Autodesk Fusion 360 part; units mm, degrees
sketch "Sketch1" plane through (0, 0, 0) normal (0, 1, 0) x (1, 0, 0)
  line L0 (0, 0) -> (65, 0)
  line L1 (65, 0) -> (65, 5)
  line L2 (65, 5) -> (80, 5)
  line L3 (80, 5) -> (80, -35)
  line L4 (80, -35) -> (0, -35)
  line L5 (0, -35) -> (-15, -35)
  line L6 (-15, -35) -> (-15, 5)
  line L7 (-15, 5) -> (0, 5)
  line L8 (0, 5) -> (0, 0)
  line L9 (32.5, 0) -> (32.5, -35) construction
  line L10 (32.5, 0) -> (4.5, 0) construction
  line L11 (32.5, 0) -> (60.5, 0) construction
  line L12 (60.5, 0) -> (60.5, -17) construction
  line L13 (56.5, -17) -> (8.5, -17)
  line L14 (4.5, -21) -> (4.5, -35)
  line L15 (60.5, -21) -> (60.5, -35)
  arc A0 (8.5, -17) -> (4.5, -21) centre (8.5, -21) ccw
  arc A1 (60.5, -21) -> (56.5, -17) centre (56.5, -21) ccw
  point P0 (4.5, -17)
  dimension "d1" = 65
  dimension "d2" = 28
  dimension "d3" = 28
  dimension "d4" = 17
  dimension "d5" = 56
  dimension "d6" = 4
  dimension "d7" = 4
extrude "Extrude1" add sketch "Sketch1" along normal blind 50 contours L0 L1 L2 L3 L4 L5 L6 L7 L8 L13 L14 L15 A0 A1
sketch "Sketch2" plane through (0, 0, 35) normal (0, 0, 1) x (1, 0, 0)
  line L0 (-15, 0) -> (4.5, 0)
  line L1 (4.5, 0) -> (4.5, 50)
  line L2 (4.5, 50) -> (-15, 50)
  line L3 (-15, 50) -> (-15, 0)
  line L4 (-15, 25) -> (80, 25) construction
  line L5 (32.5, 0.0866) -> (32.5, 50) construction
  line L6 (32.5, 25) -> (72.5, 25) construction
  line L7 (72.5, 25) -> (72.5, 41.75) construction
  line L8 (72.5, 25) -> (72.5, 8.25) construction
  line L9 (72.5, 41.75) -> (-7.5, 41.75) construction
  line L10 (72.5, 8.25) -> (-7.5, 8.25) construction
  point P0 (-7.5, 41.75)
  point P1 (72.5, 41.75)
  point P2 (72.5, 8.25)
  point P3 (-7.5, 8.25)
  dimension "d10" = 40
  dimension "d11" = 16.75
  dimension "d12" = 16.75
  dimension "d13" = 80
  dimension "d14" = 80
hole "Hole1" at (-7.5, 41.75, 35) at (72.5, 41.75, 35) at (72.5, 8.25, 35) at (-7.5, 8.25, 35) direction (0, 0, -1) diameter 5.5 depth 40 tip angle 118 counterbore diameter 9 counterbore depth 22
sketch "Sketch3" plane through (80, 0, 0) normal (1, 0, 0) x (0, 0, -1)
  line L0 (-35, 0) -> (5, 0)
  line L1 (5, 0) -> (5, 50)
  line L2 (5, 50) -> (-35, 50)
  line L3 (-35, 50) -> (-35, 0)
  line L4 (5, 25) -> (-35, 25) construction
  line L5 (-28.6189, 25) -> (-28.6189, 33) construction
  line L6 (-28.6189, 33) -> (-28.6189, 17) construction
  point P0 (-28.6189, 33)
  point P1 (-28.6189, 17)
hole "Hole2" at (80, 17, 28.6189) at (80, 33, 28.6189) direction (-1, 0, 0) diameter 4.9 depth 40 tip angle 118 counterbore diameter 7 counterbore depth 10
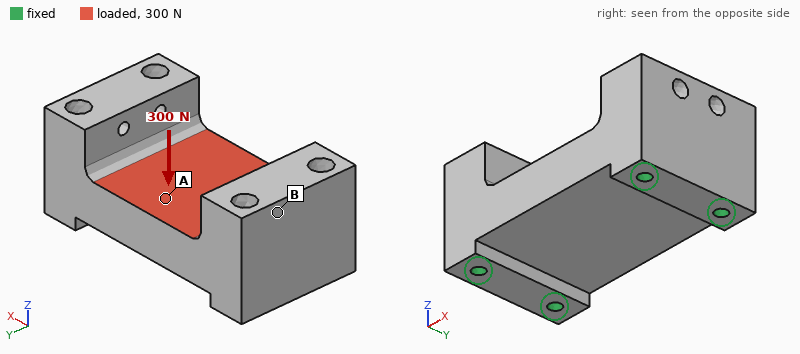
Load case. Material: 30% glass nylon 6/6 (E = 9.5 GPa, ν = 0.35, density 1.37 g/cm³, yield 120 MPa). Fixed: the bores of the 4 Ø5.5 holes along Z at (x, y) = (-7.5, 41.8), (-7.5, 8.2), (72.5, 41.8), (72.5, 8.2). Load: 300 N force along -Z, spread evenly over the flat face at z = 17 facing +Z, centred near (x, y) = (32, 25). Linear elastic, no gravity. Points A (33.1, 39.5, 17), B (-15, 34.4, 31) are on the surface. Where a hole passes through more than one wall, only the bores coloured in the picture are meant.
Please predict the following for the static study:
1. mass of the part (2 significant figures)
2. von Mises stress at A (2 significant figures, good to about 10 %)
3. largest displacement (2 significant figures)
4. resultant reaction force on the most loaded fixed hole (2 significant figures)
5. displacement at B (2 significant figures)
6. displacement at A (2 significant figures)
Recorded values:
160 g
0.69 MPa
5.3 µm
83 N
2.8 µm
4.9 µm
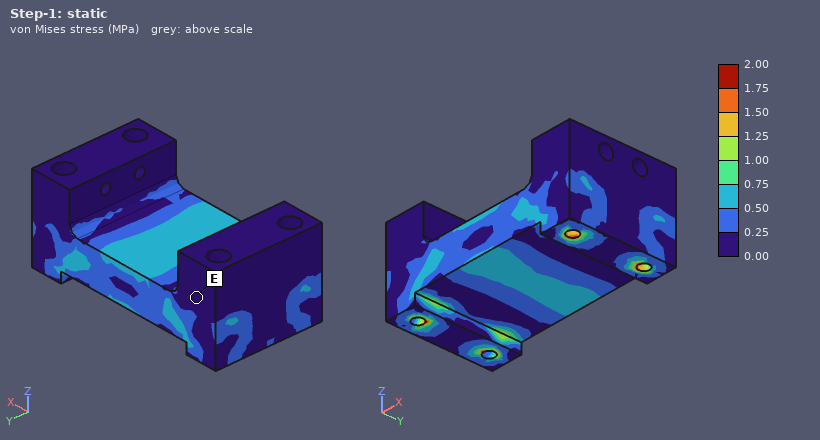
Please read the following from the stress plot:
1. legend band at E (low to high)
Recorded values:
0.00 to 0.25 MPa
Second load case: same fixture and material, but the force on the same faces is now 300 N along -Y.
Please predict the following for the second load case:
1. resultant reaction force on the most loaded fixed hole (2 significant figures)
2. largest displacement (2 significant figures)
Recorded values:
110 N
3.6 µm
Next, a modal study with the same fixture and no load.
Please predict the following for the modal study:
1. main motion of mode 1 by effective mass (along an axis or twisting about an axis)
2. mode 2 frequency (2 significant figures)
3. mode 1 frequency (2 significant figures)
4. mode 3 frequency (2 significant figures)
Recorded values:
along Z
7300 Hz
4700 Hz
7500 Hz
